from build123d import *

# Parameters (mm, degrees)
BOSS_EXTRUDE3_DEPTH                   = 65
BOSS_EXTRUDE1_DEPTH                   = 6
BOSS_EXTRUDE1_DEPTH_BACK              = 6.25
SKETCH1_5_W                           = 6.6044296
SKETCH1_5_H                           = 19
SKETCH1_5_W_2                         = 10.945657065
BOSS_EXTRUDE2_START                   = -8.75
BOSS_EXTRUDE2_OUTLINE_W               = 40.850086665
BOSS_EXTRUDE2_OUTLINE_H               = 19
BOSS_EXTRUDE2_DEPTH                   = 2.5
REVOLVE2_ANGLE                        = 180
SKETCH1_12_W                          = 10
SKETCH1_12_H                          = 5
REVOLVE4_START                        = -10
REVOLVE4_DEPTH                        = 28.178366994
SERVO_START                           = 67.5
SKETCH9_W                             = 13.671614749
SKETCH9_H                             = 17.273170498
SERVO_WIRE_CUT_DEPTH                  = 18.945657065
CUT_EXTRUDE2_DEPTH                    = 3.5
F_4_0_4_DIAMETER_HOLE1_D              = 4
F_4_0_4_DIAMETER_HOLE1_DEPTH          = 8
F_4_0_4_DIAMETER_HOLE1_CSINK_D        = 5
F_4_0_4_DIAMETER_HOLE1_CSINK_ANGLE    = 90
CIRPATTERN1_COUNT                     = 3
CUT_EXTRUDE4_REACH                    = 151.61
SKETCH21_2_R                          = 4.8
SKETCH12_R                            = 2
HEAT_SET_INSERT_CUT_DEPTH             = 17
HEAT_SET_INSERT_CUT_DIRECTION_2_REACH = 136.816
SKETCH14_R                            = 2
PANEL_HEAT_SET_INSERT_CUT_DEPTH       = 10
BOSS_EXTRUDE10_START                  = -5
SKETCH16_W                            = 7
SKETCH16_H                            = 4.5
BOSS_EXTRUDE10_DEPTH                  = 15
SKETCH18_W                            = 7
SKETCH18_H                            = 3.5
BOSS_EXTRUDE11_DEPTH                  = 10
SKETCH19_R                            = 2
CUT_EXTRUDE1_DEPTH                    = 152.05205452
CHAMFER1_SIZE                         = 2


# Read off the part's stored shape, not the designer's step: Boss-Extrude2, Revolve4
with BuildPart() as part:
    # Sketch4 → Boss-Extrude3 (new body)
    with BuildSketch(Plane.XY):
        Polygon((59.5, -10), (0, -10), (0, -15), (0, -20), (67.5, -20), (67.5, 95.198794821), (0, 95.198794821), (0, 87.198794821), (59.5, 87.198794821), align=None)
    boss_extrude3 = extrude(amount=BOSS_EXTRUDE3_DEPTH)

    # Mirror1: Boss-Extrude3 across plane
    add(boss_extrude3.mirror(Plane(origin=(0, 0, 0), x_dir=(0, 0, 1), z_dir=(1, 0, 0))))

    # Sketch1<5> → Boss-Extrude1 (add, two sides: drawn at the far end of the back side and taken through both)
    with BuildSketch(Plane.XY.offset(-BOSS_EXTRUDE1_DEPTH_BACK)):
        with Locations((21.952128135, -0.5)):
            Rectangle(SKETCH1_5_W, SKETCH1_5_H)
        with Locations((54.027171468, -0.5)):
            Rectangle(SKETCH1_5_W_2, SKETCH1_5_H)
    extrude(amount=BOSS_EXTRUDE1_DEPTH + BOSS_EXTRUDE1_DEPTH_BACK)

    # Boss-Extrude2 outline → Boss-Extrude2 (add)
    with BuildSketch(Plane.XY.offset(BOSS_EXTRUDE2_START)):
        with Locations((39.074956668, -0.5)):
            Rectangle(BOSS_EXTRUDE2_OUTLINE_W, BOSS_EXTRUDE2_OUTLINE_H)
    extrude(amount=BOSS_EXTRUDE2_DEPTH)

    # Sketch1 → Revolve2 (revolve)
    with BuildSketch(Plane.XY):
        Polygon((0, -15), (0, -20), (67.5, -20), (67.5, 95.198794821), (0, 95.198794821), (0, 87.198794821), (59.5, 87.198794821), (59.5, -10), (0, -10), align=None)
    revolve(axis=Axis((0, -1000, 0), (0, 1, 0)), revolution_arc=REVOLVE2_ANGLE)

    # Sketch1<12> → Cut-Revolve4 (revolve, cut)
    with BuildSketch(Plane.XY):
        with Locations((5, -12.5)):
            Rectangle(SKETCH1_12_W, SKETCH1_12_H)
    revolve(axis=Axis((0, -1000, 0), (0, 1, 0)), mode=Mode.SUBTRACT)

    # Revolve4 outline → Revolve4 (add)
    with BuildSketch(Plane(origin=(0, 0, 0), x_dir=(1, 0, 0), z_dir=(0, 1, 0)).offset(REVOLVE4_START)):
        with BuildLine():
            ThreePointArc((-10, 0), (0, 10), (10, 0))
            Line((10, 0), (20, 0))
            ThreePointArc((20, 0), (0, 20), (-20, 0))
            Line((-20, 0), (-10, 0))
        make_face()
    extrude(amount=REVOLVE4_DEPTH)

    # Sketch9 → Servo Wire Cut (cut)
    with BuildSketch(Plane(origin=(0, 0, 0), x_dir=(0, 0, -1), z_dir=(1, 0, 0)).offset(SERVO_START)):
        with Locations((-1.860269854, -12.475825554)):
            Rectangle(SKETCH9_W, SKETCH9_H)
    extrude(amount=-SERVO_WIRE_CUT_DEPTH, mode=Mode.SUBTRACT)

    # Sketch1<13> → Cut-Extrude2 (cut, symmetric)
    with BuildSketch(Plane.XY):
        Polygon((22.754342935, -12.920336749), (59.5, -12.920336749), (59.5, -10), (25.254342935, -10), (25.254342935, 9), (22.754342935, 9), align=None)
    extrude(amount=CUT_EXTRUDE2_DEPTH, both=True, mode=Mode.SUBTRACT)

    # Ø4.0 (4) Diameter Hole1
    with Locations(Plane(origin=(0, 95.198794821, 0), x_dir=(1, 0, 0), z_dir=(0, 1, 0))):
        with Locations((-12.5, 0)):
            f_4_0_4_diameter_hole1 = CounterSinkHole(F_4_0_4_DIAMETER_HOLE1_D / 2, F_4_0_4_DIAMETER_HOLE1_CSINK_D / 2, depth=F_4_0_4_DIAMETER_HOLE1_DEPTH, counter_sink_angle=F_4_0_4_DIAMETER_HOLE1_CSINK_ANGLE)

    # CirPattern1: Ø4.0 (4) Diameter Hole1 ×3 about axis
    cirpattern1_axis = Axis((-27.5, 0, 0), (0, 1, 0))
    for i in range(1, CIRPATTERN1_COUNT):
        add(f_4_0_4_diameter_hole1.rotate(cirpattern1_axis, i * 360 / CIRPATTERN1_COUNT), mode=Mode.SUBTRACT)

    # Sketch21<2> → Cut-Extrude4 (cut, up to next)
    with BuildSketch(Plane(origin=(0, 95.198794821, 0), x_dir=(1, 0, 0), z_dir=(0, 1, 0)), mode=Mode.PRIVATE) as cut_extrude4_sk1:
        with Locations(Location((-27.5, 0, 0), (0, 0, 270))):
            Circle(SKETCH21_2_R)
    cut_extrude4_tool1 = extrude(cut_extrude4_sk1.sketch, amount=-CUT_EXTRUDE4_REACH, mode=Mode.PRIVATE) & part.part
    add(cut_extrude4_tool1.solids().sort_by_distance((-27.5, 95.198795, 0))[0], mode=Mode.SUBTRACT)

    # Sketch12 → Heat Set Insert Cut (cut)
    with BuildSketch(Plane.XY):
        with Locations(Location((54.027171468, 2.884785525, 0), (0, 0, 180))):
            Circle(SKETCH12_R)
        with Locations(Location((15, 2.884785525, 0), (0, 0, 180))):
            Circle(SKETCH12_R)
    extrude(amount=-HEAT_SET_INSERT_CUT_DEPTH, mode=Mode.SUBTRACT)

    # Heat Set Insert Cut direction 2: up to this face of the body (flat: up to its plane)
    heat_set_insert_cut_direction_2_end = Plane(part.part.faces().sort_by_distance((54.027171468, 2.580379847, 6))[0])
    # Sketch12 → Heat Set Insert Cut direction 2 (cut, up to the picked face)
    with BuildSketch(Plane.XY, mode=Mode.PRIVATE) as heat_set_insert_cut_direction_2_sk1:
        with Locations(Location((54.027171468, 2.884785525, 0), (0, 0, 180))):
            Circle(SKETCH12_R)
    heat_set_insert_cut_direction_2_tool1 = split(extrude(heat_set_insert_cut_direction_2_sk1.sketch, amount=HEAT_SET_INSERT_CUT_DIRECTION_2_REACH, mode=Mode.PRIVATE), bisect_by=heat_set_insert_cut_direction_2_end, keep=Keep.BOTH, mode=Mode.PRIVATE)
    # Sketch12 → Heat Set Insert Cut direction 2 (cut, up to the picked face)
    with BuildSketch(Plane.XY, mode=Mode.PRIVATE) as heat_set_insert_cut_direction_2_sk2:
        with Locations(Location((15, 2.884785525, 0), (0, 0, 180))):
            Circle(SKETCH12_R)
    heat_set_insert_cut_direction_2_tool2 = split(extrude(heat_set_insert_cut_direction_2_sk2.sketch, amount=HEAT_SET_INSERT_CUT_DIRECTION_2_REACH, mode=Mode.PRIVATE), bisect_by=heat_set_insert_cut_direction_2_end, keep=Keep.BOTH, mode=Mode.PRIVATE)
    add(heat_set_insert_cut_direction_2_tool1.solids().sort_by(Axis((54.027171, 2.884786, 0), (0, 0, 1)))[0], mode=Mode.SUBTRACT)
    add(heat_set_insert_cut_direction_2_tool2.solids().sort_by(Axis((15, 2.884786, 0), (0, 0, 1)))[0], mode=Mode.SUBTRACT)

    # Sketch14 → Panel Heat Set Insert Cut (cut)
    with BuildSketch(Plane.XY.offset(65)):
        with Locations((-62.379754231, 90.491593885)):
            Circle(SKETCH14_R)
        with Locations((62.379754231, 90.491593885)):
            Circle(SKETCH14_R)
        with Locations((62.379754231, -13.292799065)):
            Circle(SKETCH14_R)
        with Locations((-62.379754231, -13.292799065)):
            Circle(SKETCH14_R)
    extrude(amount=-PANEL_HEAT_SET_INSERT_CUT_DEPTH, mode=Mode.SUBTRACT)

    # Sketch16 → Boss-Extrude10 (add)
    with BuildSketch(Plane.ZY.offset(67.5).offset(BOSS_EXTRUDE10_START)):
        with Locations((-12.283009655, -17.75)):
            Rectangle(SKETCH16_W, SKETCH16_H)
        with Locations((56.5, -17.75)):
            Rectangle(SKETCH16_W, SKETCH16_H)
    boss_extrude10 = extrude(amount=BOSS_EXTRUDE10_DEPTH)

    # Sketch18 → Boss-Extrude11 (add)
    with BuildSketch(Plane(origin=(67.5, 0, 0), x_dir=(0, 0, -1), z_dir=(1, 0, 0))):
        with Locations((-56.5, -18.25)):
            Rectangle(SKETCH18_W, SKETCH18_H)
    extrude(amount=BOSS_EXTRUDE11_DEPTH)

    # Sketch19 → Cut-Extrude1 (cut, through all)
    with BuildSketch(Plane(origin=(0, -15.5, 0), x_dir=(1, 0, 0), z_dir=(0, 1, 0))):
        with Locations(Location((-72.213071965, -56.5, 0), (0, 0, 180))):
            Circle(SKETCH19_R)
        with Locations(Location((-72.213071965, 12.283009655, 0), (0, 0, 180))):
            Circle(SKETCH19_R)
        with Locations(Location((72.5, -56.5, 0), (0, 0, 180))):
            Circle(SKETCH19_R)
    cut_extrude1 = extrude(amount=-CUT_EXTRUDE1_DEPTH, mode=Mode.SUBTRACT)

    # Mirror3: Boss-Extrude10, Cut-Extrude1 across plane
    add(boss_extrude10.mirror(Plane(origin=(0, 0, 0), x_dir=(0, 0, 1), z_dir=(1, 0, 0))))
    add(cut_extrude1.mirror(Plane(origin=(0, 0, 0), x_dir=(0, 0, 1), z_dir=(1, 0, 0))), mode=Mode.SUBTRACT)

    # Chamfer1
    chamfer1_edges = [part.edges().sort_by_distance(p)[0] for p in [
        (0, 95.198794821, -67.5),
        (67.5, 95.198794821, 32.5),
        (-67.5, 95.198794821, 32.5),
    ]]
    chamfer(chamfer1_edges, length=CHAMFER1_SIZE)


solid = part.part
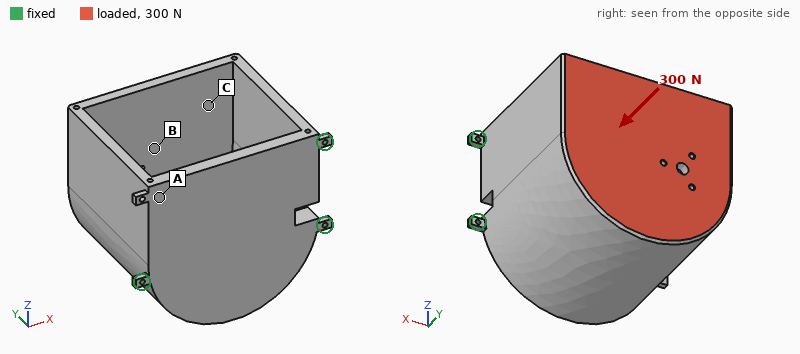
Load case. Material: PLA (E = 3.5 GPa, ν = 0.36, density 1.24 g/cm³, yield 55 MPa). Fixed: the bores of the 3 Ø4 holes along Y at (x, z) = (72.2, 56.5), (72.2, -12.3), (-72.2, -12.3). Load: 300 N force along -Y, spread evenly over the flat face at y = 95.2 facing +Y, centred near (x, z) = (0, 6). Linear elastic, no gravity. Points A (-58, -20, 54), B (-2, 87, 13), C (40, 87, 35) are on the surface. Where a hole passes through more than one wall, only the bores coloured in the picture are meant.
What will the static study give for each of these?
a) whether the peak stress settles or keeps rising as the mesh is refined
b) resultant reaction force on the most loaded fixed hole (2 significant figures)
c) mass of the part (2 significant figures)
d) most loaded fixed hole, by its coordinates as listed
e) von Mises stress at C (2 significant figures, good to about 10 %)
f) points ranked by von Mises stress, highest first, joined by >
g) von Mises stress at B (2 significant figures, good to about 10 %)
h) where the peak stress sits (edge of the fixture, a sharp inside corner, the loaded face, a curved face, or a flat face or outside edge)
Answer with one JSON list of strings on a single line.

["keeps rising", "160 N", "690 g", "(-72.2, -12.3)", "0.49 MPa", "B > C > A", "1.1 MPa", "edge of the fixture"]
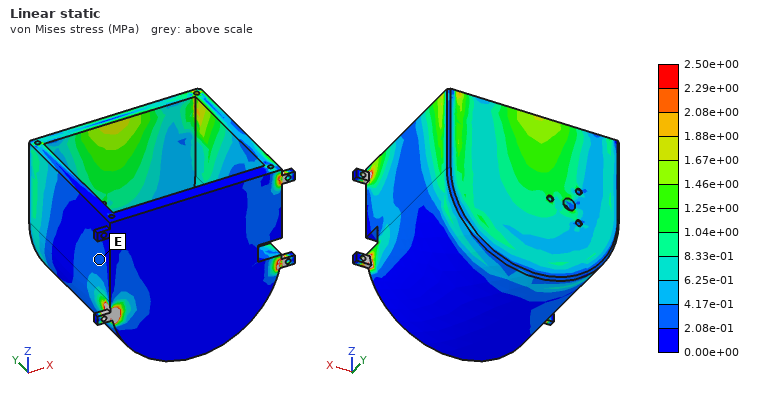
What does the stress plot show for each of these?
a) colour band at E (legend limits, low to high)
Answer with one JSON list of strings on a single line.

["2.08e-01 to 4.17e-01 MPa"]
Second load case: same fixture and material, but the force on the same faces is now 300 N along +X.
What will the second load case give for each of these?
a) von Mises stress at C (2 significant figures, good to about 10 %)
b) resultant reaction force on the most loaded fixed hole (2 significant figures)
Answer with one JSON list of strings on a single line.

["2.2 MPa", "270 N"]
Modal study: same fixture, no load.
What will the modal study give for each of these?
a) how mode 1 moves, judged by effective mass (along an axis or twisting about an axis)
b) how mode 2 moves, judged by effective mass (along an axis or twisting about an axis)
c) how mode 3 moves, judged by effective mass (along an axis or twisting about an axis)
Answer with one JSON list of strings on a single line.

["along Z", "along X", "along Y"]
